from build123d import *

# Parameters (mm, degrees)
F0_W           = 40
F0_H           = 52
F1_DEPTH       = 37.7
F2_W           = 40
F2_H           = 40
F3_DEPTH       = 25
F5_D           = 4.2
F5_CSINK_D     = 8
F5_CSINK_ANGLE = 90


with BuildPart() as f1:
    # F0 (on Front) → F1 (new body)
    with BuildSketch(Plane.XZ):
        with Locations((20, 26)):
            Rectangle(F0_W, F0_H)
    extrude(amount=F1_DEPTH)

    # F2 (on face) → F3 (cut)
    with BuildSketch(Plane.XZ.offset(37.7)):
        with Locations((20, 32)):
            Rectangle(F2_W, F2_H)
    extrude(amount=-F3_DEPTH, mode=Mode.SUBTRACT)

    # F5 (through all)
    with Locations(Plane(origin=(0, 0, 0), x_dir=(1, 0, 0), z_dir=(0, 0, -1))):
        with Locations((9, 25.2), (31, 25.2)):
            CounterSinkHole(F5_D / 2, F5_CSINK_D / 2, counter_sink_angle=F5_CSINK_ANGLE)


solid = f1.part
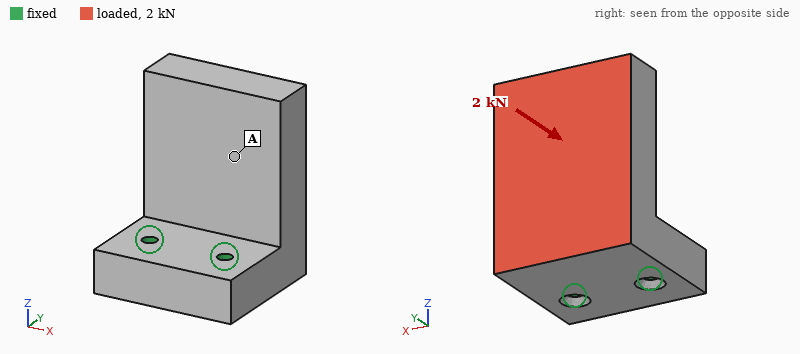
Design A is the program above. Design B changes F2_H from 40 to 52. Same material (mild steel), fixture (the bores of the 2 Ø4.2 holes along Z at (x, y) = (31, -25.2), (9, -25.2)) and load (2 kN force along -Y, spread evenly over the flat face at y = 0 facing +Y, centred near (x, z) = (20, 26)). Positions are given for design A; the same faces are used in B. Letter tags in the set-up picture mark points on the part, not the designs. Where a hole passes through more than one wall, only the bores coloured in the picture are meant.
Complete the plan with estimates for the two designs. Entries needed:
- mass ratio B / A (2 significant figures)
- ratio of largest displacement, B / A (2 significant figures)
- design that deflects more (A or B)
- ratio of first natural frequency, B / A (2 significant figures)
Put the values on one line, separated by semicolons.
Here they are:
0.85; 6.7; B; 0.38
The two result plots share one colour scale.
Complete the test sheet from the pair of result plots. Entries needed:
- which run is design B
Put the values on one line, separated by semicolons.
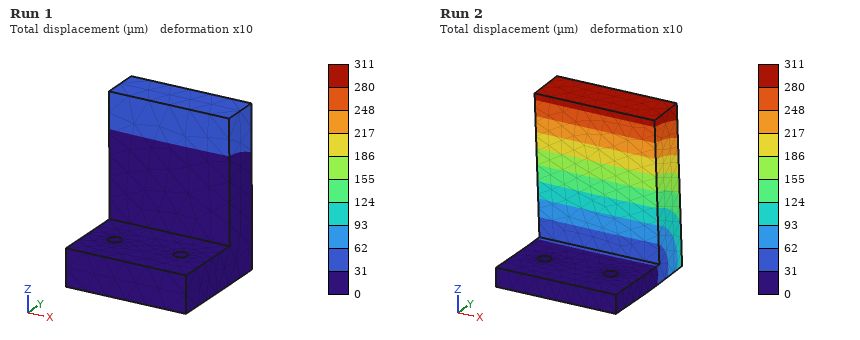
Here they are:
Run 2
